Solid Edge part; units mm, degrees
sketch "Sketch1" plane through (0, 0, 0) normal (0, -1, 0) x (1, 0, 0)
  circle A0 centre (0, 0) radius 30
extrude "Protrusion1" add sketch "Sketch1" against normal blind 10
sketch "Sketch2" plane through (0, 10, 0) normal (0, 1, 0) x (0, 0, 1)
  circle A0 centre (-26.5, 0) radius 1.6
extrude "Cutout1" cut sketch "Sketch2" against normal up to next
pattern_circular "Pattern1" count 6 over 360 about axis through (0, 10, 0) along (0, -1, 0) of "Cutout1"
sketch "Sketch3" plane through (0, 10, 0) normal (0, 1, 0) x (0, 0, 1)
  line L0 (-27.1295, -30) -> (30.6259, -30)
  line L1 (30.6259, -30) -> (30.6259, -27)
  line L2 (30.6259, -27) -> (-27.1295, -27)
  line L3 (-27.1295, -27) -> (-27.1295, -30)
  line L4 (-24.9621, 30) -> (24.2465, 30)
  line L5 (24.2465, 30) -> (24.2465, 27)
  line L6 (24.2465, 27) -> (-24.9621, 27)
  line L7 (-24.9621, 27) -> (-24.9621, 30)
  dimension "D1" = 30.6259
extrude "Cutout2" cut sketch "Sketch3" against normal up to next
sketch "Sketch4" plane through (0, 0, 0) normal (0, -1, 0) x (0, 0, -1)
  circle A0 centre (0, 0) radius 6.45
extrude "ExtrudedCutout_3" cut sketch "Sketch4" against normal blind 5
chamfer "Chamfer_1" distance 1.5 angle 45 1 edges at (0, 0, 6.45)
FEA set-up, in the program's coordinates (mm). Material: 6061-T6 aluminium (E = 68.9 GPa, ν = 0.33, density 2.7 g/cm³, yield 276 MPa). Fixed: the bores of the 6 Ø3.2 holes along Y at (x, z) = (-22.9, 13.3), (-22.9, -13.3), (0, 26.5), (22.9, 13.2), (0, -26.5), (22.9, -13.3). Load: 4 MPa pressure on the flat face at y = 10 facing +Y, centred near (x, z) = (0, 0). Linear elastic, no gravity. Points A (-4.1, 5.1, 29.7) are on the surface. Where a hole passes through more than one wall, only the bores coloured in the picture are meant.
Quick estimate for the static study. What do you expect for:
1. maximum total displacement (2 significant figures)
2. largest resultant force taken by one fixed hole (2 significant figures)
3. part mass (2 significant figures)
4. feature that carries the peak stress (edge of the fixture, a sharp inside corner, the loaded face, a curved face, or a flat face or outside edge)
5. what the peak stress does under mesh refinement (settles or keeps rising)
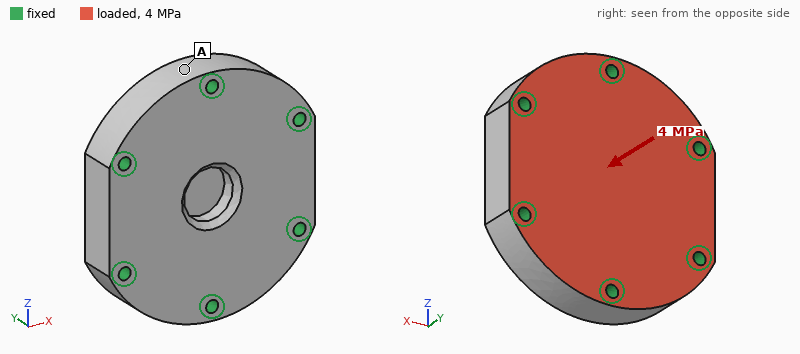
15 µm
1.9 kN
70 g
edge of the fixture
keeps rising
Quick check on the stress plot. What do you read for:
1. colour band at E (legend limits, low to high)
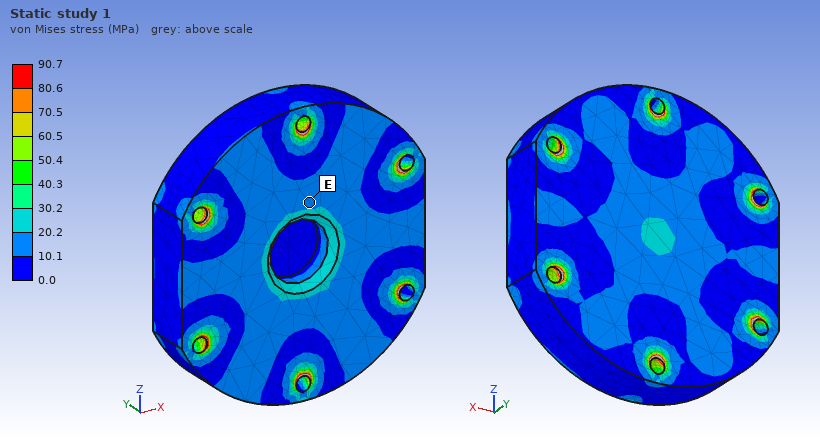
10.1 to 20.2 MPa
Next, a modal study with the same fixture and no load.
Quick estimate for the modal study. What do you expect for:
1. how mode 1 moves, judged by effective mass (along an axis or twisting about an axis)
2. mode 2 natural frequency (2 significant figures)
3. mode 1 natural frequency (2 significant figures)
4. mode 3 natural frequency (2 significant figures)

along Y
36 kHz
21 kHz
36 kHz
